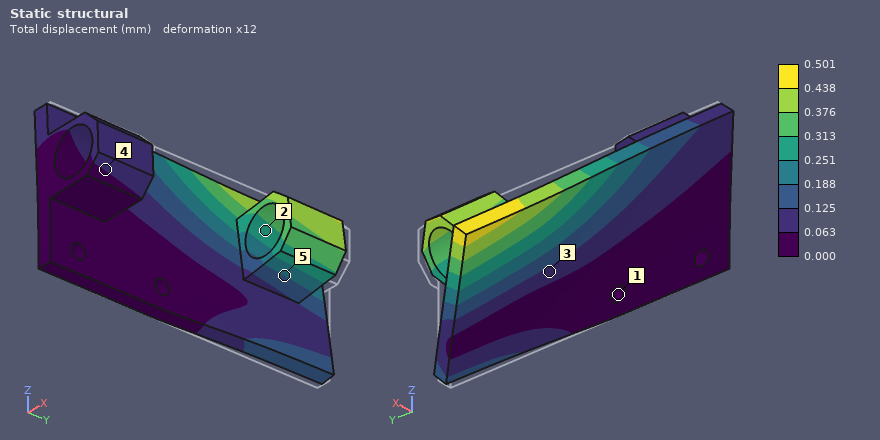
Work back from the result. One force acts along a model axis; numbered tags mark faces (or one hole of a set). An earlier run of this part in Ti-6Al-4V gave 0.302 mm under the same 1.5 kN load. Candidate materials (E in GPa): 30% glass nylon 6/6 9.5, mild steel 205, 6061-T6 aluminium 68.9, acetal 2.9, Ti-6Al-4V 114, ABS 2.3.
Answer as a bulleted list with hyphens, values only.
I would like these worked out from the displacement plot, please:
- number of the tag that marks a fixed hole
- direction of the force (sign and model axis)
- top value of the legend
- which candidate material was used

- 1
- +Z
- 0.501 mm
- 6061-T6 aluminium
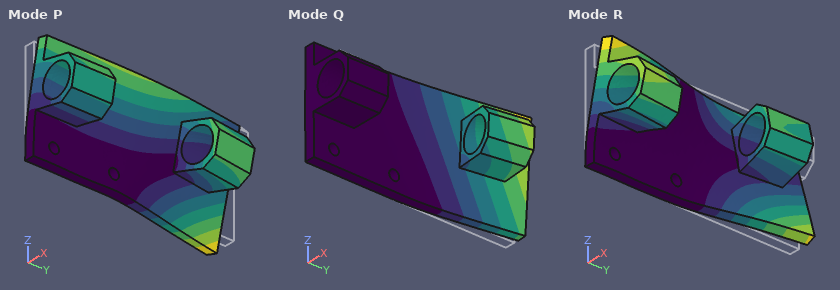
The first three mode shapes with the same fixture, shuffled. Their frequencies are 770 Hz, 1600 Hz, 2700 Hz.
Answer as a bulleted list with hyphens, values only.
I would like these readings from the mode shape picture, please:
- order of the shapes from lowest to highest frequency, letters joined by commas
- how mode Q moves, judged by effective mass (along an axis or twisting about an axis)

- Q, P, R
- along X
